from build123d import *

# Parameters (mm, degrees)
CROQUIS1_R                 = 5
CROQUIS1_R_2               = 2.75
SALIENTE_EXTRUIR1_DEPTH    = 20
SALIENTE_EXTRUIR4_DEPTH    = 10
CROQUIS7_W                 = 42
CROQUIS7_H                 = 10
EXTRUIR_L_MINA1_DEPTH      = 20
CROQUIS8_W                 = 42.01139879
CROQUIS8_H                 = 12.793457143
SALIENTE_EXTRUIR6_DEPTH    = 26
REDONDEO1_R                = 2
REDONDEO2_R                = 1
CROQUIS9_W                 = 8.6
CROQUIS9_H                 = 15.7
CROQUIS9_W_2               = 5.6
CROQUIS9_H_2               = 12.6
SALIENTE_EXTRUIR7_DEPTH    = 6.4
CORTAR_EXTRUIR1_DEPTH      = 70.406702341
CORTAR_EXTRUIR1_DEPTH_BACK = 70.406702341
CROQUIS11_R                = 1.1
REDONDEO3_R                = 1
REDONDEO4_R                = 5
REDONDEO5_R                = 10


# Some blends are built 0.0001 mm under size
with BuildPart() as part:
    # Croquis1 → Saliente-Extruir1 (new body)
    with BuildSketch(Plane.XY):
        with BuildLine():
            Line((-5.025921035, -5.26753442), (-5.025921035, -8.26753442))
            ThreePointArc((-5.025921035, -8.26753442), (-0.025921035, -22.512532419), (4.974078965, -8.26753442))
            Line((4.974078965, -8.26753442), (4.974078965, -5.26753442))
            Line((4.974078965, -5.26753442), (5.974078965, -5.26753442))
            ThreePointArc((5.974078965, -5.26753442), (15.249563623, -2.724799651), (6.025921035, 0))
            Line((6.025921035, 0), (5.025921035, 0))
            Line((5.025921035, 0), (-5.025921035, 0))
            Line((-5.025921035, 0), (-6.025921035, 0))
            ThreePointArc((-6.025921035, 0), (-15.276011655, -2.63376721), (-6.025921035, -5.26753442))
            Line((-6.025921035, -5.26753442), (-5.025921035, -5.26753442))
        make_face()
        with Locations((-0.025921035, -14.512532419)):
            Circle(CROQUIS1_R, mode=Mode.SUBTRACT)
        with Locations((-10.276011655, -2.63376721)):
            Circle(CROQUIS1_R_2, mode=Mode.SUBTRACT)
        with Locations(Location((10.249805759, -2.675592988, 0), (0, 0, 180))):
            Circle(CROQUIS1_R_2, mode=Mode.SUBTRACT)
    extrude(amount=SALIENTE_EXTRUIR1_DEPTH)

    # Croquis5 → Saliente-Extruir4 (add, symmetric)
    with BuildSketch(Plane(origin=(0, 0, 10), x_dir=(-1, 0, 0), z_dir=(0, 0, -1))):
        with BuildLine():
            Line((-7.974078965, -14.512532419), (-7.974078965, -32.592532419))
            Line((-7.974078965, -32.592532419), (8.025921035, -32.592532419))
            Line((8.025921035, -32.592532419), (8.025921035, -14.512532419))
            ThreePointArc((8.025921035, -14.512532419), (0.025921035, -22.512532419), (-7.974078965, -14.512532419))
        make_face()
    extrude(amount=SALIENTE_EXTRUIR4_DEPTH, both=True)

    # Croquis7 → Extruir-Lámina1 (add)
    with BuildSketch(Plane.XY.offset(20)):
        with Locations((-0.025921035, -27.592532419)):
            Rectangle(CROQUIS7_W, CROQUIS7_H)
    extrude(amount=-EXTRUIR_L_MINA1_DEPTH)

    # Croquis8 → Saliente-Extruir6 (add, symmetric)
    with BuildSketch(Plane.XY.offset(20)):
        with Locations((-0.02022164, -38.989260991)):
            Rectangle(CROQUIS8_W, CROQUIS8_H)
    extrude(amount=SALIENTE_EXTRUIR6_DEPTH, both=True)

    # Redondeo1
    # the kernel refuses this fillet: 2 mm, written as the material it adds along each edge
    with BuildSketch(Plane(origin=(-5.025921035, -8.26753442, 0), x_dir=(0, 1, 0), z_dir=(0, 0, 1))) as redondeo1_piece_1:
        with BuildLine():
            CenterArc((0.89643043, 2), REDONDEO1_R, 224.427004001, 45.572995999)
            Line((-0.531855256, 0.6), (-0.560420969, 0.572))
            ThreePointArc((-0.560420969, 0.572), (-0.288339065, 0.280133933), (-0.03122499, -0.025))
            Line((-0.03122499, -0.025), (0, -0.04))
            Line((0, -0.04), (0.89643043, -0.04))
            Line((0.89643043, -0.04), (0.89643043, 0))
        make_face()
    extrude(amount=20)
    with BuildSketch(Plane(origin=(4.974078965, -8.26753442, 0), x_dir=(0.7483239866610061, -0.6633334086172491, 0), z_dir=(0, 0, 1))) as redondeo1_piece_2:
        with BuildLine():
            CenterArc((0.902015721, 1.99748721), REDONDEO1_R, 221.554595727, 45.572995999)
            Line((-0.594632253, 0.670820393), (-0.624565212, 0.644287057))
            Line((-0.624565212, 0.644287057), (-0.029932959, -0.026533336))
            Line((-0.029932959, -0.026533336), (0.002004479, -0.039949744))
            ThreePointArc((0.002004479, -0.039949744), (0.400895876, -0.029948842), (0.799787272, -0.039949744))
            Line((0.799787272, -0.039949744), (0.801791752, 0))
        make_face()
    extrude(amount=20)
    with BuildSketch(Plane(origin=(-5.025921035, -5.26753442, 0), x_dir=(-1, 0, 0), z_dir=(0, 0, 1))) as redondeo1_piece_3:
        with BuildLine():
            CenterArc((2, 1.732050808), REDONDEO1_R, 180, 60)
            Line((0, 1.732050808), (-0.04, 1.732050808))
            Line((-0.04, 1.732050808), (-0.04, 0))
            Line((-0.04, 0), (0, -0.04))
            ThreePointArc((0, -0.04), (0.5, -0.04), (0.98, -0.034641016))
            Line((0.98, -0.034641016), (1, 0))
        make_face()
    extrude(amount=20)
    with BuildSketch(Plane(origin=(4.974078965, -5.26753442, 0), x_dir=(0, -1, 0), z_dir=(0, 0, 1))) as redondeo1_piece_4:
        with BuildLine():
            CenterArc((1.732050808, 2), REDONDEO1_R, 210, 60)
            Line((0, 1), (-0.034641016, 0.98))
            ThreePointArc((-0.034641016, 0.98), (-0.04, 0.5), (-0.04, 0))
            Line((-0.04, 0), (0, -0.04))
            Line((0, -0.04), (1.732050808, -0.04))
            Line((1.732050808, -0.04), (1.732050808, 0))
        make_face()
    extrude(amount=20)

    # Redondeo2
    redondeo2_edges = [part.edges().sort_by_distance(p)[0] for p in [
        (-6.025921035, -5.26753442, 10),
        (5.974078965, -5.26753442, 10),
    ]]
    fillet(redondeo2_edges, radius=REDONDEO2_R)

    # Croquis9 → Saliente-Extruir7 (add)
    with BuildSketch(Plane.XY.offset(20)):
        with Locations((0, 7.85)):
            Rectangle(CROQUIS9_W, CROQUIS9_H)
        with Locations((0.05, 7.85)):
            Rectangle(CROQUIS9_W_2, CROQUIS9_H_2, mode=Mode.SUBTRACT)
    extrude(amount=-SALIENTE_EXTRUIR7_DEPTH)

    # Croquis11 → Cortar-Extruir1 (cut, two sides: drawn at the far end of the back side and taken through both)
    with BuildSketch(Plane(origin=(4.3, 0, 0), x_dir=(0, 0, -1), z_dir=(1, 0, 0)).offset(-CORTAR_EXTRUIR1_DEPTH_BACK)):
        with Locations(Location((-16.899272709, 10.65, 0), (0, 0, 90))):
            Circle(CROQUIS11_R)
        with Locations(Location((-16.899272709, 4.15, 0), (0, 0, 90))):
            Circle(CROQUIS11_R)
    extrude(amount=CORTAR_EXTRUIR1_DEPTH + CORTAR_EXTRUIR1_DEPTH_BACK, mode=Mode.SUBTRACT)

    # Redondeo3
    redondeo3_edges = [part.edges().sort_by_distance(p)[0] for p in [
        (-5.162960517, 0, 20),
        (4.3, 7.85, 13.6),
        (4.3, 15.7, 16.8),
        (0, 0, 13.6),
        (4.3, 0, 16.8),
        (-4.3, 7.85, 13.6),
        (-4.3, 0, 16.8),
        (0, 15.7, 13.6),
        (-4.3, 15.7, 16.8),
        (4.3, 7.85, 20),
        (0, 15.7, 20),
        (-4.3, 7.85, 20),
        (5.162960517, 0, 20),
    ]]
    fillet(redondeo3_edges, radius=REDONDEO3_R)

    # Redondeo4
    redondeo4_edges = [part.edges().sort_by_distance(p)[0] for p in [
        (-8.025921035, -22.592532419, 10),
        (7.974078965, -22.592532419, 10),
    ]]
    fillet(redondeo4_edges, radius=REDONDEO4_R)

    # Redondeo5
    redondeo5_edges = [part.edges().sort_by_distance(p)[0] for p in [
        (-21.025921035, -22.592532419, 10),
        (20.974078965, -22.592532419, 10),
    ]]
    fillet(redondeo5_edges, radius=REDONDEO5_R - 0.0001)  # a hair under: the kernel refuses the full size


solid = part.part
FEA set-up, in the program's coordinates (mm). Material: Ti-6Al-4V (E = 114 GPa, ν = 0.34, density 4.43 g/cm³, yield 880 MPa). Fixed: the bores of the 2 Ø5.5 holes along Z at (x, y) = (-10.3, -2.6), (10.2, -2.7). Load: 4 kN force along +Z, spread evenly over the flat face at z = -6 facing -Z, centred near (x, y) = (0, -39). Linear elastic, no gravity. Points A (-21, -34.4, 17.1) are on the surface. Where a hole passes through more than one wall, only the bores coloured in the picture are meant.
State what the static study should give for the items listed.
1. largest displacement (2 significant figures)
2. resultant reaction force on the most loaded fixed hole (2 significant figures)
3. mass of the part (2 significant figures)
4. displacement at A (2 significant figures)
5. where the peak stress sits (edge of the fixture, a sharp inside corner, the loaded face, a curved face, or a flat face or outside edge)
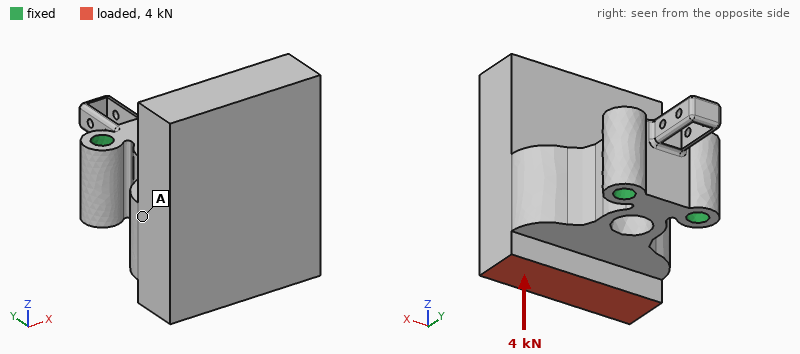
0.36 mm
2.0 kN
190 g
0.19 mm
a curved face
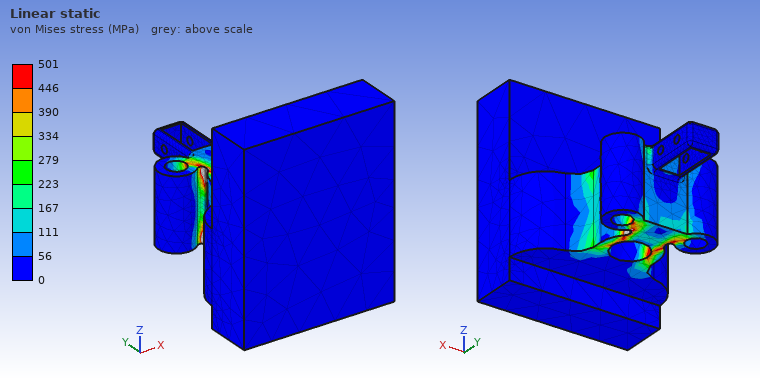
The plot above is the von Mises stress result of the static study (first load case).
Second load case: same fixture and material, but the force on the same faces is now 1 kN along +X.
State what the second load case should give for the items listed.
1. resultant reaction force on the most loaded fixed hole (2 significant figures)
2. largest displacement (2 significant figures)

2.7 kN
0.15 mm
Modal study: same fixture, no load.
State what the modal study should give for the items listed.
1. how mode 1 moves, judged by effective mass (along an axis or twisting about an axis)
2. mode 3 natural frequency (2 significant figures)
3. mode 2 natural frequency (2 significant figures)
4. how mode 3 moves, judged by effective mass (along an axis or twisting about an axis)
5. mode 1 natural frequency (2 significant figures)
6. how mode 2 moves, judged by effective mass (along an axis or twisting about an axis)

along X
2500 Hz
1600 Hz
twisting about Y
1200 Hz
along Z
